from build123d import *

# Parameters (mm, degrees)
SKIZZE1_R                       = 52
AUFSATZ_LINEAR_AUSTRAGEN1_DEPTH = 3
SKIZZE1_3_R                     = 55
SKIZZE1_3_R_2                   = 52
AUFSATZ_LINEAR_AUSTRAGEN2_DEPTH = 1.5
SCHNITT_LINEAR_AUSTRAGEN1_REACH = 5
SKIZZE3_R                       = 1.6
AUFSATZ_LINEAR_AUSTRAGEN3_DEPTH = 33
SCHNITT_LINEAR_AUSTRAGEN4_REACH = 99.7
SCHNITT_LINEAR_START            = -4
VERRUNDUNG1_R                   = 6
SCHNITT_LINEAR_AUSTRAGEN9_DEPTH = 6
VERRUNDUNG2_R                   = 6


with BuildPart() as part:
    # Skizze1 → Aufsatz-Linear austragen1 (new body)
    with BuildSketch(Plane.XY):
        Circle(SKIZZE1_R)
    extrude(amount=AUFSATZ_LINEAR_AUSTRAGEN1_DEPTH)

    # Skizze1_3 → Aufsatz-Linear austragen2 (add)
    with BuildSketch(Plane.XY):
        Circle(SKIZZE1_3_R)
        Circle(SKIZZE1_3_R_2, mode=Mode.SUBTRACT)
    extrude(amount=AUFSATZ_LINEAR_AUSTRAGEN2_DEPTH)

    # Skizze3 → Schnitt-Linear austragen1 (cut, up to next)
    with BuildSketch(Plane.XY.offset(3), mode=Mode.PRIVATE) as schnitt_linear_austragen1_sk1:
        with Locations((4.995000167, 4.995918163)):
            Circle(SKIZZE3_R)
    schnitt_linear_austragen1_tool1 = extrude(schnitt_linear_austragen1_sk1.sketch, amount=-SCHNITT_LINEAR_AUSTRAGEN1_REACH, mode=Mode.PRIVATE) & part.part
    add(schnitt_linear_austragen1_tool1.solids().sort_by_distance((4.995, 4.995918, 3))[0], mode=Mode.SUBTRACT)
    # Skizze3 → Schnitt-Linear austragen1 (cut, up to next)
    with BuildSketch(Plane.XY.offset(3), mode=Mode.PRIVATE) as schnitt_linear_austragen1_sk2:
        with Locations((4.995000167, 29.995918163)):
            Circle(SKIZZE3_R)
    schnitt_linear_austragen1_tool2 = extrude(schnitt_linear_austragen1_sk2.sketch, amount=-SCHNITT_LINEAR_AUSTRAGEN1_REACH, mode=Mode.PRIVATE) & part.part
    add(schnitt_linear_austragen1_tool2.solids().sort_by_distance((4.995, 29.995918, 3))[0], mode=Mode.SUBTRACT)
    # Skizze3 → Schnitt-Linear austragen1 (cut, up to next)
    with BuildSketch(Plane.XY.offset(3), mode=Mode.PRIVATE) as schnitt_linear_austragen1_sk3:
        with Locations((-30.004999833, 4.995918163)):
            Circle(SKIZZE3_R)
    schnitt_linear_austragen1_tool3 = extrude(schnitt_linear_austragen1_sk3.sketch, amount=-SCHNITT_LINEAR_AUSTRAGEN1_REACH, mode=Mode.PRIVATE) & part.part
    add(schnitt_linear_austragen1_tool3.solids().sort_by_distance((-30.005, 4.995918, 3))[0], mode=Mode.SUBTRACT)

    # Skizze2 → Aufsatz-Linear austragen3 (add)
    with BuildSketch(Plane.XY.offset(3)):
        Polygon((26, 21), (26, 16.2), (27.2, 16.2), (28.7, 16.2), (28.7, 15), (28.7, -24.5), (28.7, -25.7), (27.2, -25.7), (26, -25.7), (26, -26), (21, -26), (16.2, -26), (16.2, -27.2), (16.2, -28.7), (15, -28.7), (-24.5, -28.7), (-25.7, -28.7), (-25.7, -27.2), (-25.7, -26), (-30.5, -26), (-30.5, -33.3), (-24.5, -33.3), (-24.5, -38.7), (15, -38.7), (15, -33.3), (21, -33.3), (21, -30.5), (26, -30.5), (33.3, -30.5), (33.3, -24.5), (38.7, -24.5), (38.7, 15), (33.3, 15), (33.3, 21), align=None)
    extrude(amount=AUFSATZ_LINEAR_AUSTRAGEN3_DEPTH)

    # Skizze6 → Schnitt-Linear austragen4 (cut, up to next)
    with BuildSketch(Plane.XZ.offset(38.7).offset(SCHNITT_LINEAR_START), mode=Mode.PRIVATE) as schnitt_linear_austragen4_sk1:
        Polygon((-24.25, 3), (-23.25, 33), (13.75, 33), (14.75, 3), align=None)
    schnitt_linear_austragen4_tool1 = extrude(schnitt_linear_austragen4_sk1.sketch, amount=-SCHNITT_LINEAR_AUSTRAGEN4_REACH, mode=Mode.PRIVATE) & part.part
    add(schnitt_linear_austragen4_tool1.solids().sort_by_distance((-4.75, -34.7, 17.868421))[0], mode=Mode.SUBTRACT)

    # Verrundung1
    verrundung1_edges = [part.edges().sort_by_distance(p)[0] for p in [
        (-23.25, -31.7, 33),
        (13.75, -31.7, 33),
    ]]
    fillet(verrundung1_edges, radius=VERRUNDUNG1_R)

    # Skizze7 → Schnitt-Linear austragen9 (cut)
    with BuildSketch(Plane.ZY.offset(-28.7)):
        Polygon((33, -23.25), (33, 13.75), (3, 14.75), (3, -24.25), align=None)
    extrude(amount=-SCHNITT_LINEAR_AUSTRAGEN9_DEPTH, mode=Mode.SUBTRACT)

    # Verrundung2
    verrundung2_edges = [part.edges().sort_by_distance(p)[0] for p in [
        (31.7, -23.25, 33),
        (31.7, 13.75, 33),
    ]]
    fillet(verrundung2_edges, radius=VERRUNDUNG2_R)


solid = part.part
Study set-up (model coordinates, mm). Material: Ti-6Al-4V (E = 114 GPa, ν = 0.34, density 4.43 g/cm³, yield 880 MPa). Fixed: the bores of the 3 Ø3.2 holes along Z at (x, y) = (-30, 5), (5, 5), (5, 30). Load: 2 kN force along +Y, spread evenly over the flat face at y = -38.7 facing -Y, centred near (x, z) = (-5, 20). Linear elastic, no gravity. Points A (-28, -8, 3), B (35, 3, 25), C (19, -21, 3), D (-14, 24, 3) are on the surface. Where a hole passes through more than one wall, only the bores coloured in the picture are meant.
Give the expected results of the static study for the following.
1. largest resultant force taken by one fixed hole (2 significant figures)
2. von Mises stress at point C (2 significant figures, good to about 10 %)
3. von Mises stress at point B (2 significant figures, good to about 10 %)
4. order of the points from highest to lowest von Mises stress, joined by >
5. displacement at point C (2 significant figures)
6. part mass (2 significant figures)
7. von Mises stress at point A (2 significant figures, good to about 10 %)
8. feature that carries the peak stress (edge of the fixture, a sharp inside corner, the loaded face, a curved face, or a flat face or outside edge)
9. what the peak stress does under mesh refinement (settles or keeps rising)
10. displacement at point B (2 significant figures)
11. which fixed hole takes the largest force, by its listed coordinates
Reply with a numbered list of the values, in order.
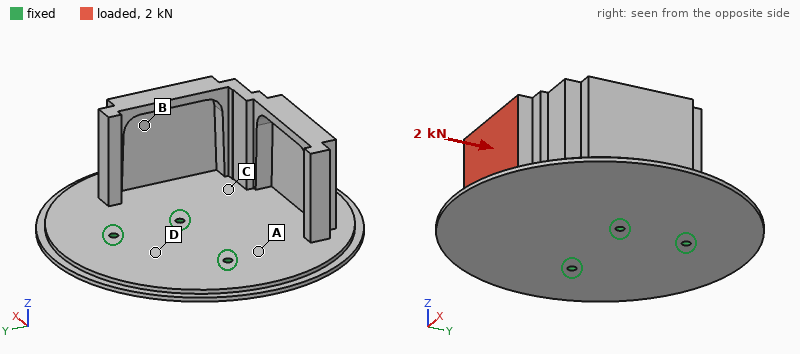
1. 1.3 kN
2. 73 MPa
3. 45 MPa
4. A > C > B > D
5. 0.41 mm
6. 200 g
7. 120 MPa
8. edge of the fixture
9. keeps rising
10. 0.40 mm
11. (5, 5)
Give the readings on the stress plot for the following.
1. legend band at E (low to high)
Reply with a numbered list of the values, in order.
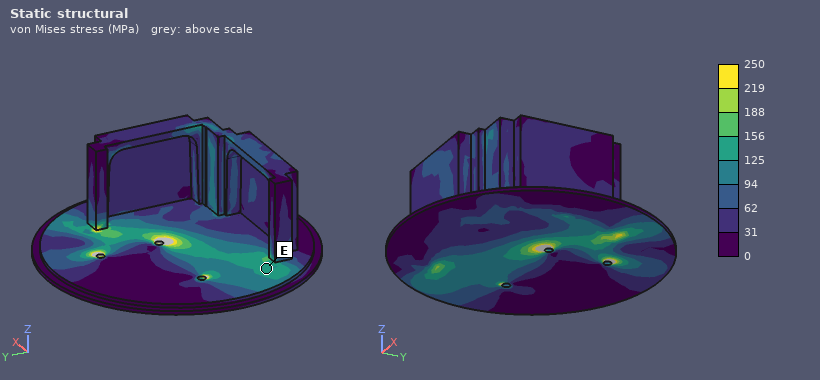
1. 125 to 156 MPa
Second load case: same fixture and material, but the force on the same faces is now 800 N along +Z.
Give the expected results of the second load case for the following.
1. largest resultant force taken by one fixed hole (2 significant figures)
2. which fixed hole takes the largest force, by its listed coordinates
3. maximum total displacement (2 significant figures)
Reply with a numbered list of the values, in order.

1. 1.3 kN
2. (5, 5)
3. 0.92 mm
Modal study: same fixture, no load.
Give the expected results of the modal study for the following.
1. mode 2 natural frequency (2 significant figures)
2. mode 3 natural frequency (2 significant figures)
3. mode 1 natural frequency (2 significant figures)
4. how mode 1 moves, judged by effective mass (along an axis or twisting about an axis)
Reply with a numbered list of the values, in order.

1. 790 Hz
2. 1800 Hz
3. 540 Hz
4. along Z
